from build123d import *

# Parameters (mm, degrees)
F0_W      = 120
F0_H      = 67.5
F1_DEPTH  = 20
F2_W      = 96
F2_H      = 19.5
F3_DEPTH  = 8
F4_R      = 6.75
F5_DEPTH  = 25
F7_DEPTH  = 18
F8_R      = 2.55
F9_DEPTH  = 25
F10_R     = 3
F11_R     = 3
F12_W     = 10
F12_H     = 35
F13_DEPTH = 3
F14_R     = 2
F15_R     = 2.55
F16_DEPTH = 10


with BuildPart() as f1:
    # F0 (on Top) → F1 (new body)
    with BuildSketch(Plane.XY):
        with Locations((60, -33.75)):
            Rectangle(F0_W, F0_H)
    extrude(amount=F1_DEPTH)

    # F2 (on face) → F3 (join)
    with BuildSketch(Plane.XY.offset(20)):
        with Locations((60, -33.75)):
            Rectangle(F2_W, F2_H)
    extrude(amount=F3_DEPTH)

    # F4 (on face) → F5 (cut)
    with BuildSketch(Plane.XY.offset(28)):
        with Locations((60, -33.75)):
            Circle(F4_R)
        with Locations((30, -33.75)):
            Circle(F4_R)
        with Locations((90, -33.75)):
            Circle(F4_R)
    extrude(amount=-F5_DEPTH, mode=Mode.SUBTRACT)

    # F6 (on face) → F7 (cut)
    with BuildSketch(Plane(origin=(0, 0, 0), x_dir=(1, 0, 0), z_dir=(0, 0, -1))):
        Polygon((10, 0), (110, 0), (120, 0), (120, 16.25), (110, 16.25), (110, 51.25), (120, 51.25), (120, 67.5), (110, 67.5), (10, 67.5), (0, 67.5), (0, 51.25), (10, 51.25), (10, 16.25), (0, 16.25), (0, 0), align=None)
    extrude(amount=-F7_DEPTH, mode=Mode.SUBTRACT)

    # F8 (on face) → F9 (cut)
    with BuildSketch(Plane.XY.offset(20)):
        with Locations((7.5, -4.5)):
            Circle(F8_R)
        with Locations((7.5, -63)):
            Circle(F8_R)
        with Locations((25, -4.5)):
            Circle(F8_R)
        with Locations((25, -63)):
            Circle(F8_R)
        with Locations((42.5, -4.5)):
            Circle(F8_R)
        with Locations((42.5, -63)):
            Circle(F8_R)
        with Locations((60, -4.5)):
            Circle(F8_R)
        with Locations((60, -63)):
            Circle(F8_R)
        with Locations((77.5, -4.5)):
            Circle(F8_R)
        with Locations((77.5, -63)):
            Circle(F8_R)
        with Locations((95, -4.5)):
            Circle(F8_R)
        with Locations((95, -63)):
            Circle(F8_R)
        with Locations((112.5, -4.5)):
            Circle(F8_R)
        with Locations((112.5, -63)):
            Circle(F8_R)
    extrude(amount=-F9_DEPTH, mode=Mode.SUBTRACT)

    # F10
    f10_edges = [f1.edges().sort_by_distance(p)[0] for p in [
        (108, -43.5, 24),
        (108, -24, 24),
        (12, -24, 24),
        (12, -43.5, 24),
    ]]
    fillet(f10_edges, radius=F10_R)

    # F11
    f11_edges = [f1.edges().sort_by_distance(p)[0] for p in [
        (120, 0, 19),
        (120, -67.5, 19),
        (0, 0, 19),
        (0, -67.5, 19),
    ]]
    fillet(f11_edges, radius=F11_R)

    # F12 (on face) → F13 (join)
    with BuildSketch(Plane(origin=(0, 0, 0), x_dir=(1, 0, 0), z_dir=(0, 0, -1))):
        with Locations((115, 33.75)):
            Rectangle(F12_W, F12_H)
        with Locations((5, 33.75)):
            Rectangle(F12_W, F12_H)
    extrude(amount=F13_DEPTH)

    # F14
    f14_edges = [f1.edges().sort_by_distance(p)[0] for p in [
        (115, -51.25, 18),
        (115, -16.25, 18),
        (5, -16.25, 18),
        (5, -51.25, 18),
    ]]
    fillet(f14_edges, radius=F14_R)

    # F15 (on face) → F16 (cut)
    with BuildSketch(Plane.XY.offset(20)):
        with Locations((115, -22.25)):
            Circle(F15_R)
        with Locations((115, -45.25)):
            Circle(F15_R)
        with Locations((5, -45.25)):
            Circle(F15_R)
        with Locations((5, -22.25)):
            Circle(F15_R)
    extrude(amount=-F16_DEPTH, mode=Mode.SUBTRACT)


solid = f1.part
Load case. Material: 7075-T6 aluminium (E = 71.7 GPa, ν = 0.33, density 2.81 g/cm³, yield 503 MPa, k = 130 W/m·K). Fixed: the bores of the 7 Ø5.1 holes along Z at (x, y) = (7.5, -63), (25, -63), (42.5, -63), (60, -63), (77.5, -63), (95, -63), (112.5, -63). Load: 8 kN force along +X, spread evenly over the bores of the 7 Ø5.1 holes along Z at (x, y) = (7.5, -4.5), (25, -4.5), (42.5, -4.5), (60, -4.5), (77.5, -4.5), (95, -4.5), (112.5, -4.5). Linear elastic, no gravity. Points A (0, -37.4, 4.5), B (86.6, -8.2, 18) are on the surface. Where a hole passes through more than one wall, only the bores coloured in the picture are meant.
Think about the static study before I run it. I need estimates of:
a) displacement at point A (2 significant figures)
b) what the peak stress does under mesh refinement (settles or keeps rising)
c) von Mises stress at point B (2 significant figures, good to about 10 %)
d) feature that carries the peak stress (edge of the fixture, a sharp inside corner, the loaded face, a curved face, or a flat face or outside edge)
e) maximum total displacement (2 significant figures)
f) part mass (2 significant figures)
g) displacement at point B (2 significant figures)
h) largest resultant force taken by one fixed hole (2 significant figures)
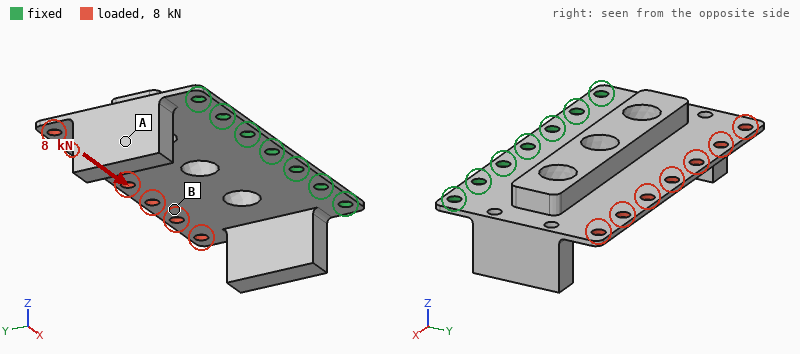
0.12 mm
keeps rising
71 MPa
edge of the fixture
0.35 mm
110 g
0.18 mm
3.5 kN
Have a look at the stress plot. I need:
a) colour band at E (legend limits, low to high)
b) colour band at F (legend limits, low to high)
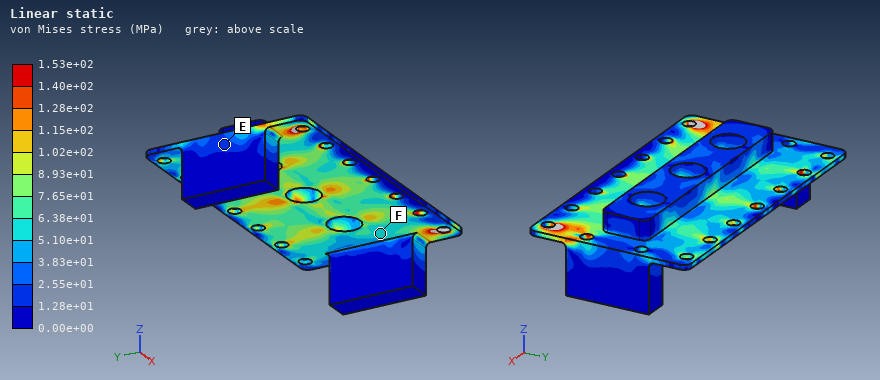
1.28e+01 to 2.55e+01 MPa
5.10e+01 to 6.38e+01 MPa
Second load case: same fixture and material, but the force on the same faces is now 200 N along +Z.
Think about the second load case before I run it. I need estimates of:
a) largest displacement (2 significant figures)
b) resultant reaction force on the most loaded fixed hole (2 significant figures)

1.4 mm
89 N
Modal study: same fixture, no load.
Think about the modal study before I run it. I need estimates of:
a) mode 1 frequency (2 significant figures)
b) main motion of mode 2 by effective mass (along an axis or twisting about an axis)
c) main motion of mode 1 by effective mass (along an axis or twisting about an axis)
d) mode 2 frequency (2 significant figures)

380 Hz
twisting about Y
along Z
1000 Hz
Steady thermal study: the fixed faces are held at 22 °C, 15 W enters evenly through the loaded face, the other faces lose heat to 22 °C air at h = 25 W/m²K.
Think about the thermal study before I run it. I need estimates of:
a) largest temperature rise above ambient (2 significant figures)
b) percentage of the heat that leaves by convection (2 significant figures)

19 K
30 %
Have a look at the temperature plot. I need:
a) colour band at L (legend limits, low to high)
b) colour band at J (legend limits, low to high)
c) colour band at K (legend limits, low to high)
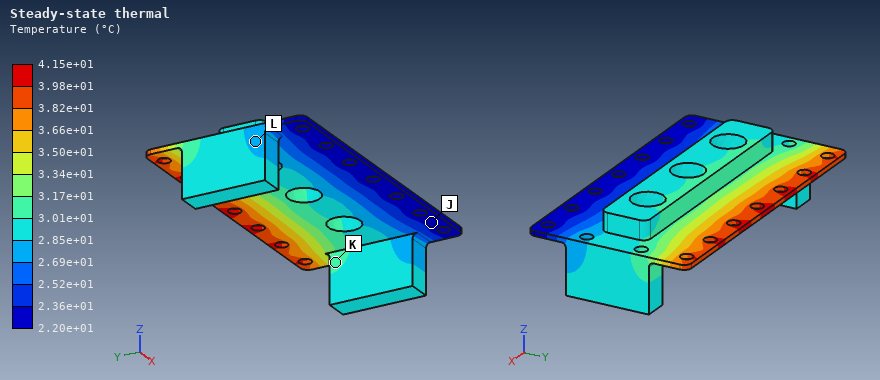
2.69e+01 to 2.85e+01 °C
2.20e+01 to 2.36e+01 °C
3.01e+01 to 3.17e+01 °C
